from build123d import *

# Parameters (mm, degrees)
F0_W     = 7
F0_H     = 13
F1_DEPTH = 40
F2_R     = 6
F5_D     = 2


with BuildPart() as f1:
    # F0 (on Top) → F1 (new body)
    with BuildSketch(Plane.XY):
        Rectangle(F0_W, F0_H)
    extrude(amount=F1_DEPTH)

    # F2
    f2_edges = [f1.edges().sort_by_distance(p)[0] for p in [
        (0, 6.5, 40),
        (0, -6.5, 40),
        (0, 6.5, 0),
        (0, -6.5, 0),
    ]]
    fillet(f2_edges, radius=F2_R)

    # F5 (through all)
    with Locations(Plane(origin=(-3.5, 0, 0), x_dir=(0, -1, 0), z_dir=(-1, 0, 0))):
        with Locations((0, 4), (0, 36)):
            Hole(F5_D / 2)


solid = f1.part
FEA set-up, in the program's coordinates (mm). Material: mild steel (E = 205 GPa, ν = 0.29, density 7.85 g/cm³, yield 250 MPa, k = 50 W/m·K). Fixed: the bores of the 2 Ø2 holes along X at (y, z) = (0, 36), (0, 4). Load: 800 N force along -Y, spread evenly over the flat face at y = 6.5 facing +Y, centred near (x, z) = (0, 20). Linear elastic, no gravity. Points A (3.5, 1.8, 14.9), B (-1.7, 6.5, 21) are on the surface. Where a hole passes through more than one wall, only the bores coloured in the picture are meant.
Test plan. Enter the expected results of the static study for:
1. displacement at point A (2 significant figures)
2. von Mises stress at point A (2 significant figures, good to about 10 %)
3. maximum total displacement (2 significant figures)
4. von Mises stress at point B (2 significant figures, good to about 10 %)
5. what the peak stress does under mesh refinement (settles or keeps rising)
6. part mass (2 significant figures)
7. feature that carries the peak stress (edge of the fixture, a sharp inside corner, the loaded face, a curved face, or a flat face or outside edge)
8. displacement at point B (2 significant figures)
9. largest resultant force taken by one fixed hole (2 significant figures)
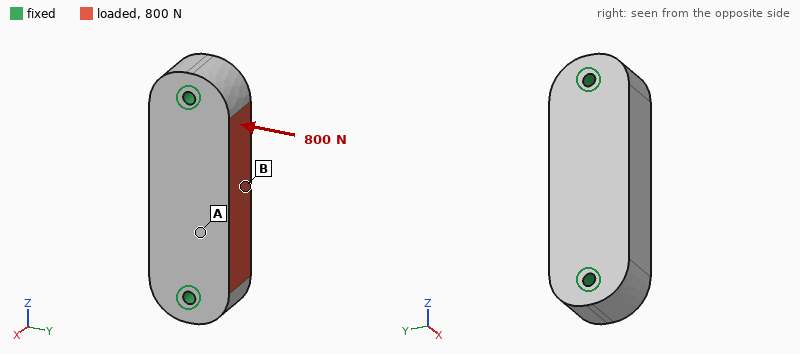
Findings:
1.4 µm
5.1 MPa
1.7 µm
14 MPa
keeps rising
27 g
edge of the fixture
1.6 µm
400 N
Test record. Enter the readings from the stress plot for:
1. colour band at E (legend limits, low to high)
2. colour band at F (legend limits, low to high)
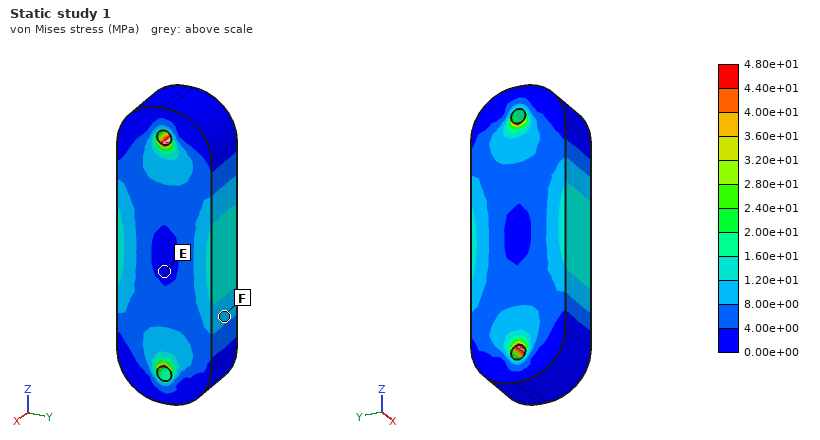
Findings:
0.00e+00 to 4.00e+00 MPa
8.00e+00 to 1.20e+01 MPa
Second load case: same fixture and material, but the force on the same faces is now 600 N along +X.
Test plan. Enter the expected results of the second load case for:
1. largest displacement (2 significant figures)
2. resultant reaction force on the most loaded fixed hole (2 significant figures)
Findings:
3.8 µm
300 N
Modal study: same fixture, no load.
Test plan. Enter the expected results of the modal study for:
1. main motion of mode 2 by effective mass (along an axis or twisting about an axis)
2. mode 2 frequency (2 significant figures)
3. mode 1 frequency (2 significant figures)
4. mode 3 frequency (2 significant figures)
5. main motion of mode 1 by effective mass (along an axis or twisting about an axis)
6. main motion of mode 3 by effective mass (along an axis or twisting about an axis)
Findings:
along Y
27 kHz
24 kHz
34 kHz
along X
twisting about Z
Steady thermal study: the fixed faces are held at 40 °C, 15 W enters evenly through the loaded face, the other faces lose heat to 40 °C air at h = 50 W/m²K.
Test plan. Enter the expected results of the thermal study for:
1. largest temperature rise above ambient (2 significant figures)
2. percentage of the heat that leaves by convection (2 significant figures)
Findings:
23 K
4.5 %
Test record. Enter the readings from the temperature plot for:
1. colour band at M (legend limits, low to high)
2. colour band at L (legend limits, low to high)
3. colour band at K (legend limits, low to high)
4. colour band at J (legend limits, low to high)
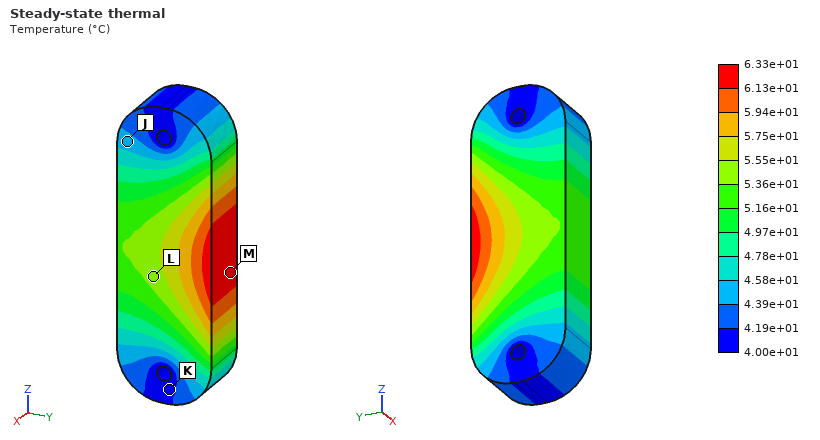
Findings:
6.13e+01 to 6.33e+01 °C
5.36e+01 to 5.55e+01 °C
4.00e+01 to 4.19e+01 °C
4.39e+01 to 4.58e+01 °C
